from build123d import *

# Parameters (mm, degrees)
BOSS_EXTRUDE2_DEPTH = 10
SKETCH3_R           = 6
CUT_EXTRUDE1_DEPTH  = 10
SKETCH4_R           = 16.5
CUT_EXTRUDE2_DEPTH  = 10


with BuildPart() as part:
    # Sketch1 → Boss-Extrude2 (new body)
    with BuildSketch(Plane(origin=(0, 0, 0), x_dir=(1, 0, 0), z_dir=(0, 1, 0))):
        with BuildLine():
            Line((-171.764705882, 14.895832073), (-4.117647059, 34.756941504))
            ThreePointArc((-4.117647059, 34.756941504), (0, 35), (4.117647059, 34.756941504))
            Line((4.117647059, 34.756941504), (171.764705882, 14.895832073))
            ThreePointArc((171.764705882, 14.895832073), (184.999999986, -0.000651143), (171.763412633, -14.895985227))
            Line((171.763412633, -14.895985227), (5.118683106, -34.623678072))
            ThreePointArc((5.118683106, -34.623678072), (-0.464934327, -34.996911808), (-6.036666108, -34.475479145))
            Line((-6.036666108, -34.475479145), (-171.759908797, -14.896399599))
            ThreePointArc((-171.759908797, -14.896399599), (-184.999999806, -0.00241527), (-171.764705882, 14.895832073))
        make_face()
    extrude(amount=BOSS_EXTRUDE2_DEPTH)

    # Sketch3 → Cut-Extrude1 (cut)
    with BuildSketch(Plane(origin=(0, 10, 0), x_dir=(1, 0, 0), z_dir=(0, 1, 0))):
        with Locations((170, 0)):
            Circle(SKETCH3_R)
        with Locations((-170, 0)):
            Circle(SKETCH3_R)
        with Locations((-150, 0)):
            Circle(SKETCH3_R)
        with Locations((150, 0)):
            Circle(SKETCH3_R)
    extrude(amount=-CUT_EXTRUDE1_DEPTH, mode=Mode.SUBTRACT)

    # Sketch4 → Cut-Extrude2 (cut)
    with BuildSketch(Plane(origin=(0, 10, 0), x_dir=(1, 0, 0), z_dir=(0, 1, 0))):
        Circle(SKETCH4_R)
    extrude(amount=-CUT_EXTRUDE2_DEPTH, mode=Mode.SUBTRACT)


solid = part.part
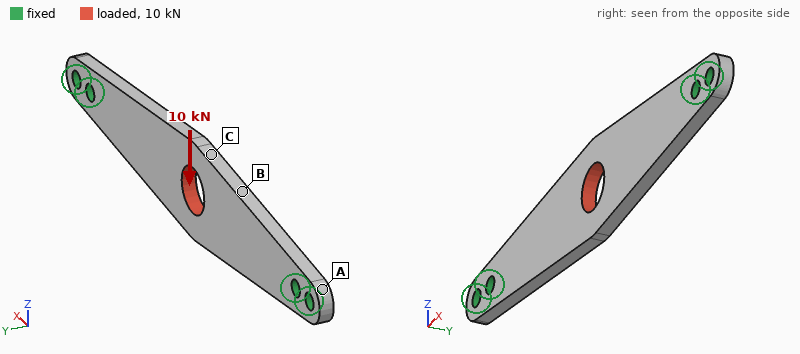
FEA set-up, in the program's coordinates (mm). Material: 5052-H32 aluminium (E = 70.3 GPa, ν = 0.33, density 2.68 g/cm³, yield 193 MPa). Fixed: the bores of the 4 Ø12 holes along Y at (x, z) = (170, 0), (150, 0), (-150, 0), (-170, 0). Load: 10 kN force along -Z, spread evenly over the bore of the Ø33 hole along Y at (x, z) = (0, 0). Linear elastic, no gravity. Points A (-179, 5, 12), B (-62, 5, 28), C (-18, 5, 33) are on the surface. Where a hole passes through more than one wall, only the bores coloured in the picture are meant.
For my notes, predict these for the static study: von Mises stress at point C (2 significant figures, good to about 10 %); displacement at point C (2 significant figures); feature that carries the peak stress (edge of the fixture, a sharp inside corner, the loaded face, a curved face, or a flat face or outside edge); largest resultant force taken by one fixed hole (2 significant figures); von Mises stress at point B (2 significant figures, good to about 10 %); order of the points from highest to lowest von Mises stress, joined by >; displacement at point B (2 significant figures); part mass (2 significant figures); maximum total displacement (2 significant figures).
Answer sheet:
71 MPa
0.26 mm
edge of the fixture
8.8 kN
46 MPa
C > B > A
0.21 mm
440 g
0.27 mm
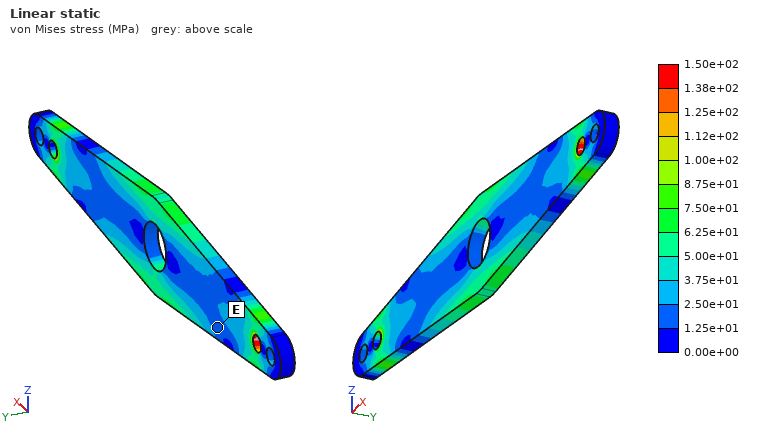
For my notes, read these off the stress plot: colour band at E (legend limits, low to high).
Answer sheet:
1.25e+01 to 2.50e+01 MPa
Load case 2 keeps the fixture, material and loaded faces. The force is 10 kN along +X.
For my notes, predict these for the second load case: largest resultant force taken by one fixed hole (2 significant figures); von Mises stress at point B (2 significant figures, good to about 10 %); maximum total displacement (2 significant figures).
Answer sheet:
4.3 kN
8.9 MPa
22 µm
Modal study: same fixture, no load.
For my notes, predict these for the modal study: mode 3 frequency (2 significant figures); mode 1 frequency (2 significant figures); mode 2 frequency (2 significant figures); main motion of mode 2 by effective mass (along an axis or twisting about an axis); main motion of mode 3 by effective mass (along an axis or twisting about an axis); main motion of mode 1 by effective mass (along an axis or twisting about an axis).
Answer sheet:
1600 Hz
540 Hz
1400 Hz
twisting about X
twisting about Z
along Y
